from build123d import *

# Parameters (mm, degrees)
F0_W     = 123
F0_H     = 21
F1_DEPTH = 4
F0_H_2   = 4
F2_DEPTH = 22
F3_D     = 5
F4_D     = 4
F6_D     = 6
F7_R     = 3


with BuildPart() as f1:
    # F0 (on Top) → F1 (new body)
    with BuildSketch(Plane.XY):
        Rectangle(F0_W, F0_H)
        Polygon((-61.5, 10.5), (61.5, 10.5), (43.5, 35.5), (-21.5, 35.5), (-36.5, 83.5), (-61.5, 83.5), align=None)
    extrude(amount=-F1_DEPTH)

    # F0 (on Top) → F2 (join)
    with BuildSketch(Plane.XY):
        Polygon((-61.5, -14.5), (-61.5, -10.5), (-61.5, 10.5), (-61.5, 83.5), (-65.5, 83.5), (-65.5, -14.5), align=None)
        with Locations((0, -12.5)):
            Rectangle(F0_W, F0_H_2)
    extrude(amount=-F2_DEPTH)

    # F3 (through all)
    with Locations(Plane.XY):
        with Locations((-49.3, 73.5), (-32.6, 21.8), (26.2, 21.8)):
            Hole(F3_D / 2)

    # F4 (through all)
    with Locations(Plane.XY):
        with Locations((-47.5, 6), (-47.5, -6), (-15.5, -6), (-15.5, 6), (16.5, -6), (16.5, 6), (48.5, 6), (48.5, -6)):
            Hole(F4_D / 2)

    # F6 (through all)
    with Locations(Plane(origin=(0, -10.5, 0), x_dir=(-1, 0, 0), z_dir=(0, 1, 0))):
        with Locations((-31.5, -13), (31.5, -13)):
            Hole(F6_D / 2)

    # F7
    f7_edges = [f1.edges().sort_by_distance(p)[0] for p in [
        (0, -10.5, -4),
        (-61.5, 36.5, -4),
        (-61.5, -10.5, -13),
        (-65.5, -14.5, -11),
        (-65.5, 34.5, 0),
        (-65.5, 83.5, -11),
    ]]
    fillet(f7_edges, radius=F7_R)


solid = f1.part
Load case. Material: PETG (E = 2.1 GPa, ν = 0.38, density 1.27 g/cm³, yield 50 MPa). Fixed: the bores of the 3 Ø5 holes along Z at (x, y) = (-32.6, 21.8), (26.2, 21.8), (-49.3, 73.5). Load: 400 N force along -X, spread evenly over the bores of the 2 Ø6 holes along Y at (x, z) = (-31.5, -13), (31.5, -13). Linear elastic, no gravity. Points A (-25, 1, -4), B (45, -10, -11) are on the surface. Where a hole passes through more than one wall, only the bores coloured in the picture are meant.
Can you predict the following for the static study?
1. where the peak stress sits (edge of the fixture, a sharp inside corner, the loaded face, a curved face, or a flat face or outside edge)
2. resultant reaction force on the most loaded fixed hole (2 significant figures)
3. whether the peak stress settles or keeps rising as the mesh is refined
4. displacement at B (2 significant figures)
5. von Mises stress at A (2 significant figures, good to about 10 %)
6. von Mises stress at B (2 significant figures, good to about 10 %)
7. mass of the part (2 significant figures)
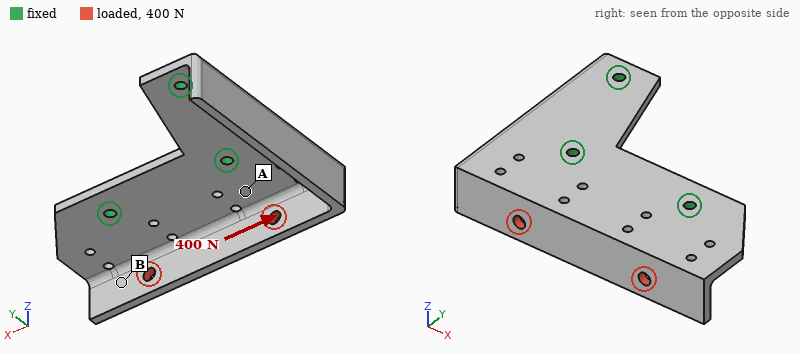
edge of the fixture
270 N
keeps rising
1.3 mm
5.6 MPa
2.0 MPa
59 g
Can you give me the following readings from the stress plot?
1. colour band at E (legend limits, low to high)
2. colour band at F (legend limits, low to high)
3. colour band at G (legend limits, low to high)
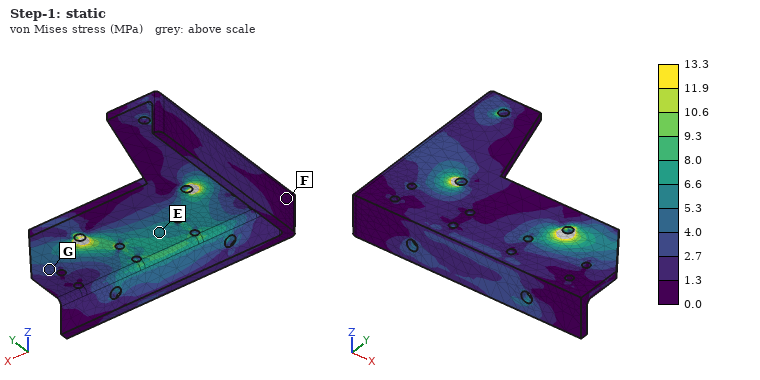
5.3 to 6.6 MPa
0.0 to 1.3 MPa
2.7 to 4.0 MPa
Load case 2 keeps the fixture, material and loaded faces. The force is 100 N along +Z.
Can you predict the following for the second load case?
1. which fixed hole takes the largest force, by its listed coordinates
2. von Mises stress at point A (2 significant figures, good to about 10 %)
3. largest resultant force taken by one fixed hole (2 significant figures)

(-32.6, 21.8)
1.9 MPa
71 N
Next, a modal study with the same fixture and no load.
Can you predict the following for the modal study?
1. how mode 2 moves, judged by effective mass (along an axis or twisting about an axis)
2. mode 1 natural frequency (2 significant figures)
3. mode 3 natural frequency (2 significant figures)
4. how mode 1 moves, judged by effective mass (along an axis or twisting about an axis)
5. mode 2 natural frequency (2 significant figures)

along Z
320 Hz
960 Hz
along Z
390 Hz
